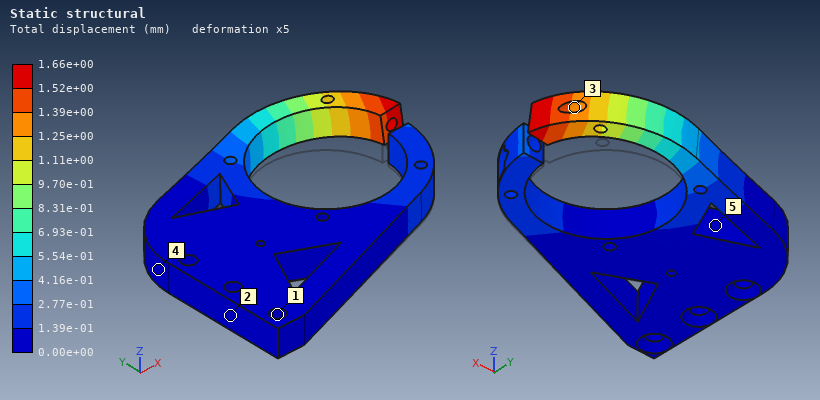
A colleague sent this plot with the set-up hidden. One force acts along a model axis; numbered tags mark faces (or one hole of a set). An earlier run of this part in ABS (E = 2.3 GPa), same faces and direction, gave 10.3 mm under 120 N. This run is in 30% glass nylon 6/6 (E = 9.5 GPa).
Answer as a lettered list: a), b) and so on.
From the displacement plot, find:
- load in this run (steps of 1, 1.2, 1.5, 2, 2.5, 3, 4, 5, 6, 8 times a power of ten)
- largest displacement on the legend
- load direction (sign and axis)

a) 80 N
b) 1.66e+00 mm
c) +Z
